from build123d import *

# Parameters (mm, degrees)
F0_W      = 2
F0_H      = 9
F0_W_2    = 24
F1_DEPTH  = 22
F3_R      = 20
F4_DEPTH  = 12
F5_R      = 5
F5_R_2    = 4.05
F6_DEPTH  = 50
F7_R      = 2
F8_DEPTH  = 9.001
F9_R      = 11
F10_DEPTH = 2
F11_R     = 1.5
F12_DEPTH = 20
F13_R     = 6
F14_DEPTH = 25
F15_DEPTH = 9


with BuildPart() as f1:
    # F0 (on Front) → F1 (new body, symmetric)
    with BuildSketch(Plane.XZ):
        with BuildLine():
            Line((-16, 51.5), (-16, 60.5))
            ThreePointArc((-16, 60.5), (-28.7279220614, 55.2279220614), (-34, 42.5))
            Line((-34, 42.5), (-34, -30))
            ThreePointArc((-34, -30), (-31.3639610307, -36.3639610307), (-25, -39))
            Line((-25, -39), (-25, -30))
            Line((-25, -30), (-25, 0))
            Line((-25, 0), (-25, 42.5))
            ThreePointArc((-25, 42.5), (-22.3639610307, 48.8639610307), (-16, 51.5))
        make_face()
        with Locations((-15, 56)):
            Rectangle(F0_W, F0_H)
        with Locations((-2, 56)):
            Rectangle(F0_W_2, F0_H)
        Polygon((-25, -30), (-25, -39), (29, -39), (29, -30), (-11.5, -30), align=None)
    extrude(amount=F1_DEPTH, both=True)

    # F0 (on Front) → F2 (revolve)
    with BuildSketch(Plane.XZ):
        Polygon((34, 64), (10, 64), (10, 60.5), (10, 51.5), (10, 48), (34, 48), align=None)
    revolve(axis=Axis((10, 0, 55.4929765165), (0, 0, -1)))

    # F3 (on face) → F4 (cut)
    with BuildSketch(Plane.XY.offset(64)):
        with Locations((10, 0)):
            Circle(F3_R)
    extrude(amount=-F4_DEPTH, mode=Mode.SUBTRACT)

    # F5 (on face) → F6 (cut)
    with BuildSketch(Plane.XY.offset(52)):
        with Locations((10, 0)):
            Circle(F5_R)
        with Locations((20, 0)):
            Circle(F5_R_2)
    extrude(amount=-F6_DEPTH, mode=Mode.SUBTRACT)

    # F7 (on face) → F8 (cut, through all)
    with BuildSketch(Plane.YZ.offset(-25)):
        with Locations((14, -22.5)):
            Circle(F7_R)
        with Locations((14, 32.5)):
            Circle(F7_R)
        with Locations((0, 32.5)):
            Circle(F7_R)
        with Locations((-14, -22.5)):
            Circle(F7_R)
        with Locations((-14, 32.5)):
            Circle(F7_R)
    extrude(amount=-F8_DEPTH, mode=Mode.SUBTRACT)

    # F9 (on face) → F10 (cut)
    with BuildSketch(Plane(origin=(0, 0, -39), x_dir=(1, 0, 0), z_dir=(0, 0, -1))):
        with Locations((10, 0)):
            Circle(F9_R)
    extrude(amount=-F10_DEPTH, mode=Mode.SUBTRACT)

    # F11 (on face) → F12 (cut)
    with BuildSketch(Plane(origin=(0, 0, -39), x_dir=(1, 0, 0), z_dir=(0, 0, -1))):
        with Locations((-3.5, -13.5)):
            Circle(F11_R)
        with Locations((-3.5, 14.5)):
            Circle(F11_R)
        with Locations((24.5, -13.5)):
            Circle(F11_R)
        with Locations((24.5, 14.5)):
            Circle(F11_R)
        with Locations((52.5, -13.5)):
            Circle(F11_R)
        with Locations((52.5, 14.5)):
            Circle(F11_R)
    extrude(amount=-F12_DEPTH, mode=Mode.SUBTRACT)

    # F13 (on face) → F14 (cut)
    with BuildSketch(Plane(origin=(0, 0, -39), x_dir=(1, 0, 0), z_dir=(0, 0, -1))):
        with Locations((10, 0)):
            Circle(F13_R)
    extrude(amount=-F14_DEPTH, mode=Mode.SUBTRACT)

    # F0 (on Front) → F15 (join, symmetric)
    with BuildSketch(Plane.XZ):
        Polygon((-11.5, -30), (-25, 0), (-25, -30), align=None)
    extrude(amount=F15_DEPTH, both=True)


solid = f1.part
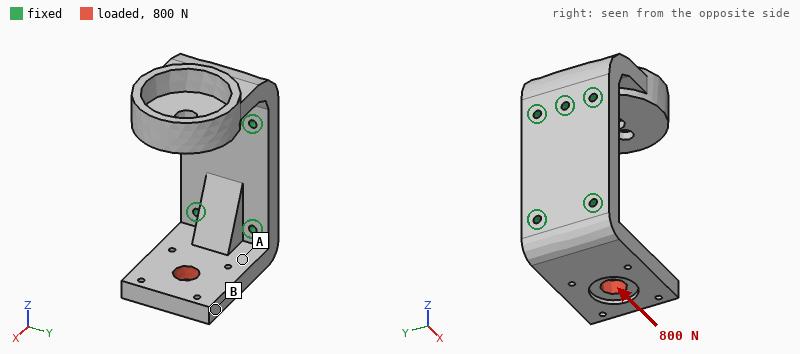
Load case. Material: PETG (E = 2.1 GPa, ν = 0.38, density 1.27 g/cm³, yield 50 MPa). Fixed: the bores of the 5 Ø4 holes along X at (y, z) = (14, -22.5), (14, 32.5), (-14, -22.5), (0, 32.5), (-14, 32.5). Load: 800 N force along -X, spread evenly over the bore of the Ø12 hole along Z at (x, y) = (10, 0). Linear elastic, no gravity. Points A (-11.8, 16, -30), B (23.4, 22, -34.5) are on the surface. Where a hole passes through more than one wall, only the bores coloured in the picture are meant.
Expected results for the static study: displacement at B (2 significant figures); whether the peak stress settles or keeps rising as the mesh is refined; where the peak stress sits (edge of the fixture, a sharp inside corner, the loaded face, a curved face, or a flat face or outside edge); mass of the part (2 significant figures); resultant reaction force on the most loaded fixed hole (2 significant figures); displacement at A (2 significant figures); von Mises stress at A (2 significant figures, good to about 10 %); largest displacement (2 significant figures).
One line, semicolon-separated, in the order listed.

0.27 mm; keeps rising; edge of the fixture; 99 g; 450 N; 0.14 mm; 2.8 MPa; 0.30 mm
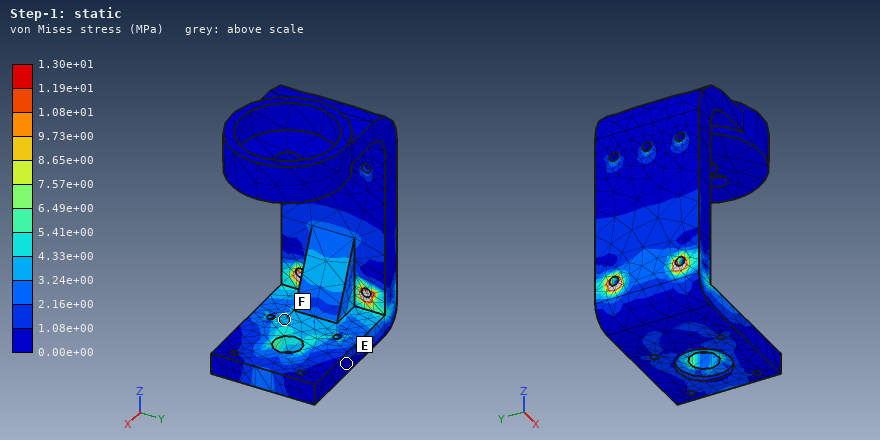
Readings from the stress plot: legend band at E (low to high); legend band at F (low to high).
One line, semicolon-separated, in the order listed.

0.00e+00 to 1.08e+00 MPa; 3.24e+00 to 4.33e+00 MPa
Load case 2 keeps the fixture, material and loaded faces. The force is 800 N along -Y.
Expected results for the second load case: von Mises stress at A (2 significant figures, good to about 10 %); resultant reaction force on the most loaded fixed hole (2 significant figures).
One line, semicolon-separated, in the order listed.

5.6 MPa; 1.1 kN
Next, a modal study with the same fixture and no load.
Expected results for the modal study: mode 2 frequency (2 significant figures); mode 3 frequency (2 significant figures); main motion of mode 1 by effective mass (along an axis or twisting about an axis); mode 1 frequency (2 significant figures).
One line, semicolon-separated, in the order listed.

660 Hz; 660 Hz; along Z; 370 Hz
